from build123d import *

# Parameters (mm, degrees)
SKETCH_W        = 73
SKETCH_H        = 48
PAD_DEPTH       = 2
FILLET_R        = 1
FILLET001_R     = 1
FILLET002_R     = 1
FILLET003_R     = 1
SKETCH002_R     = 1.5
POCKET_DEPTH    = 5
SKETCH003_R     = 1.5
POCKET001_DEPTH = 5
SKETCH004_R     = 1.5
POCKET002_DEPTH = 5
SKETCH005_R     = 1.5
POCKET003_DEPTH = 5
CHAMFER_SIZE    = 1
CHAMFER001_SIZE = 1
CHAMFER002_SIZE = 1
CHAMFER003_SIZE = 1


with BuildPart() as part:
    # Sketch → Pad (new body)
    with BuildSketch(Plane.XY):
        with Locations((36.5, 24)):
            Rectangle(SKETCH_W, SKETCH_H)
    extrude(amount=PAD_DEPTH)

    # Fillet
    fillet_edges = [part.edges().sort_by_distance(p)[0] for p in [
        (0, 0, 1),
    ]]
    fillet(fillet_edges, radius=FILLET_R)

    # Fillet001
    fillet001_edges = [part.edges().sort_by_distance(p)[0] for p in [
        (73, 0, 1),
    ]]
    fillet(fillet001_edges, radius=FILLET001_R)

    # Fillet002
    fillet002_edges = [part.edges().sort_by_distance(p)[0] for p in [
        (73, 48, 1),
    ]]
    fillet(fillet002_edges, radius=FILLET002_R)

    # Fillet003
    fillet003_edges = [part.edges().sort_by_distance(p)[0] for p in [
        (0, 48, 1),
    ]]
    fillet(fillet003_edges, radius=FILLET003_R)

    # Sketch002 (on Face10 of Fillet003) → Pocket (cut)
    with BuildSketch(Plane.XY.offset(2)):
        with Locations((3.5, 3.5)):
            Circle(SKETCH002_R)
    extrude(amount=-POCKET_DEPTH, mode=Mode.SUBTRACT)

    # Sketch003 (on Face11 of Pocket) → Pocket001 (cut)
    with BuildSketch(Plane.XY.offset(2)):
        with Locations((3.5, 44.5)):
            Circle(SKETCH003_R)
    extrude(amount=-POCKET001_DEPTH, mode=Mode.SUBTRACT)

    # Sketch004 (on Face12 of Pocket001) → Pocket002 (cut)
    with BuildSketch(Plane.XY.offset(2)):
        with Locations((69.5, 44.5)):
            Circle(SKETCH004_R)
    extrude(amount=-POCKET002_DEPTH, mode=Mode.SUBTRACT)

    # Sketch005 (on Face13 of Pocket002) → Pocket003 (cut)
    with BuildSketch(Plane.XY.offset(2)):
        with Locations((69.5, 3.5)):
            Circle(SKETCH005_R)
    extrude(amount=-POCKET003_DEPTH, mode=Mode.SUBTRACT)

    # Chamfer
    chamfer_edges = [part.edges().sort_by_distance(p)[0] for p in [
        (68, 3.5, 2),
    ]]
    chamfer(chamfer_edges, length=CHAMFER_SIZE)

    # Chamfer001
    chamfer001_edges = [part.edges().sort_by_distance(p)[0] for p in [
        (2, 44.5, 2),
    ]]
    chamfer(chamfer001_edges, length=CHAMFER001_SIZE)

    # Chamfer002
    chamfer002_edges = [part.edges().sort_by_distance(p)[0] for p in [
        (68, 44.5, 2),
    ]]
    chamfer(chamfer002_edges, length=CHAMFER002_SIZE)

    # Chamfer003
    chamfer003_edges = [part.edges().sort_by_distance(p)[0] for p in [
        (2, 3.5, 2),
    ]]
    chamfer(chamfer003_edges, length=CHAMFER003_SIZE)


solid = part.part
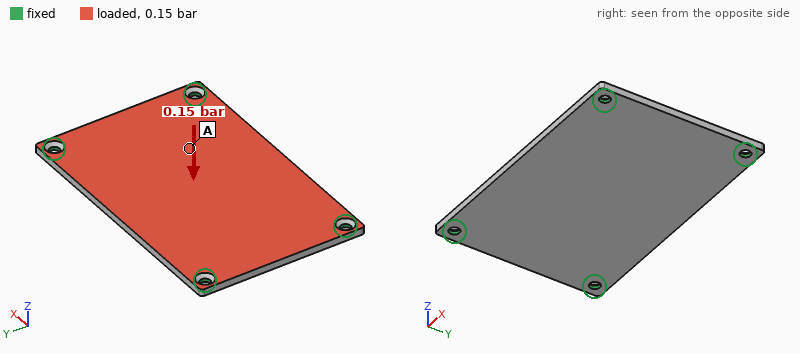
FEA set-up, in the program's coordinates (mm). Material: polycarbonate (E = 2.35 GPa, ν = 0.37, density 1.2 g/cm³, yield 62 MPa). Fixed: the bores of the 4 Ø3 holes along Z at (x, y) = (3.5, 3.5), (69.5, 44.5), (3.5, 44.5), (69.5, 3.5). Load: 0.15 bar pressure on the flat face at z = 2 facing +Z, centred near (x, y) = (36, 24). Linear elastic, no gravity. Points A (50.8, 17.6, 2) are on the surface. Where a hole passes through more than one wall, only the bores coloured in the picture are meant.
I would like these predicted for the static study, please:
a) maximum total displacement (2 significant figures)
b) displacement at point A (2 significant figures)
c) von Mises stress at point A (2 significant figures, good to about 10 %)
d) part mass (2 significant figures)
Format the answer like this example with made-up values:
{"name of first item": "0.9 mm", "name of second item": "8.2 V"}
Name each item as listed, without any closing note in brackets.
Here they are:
{"maximum total displacement": "0.80 mm", "displacement at point A": "0.61 mm", "von Mises stress at point A": "3.4 MPa", "part mass": "8.3 g"}
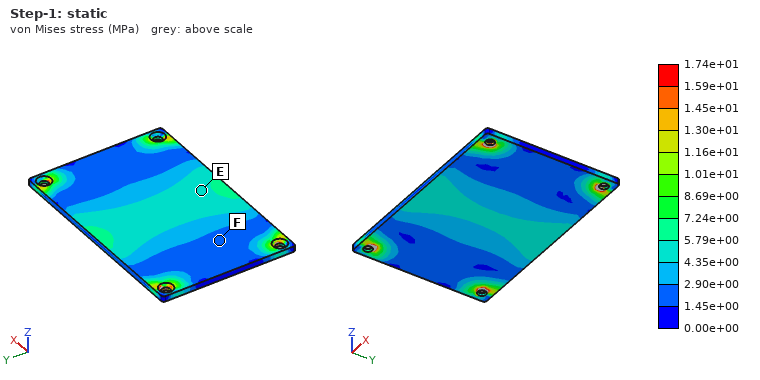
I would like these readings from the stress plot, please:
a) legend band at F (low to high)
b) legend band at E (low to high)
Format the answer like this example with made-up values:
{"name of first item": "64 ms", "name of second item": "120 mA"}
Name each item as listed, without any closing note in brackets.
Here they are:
{"legend band at F": "1.45e+00 to 2.90e+00 MPa", "legend band at E": "4.35e+00 to 5.79e+00 MPa"}
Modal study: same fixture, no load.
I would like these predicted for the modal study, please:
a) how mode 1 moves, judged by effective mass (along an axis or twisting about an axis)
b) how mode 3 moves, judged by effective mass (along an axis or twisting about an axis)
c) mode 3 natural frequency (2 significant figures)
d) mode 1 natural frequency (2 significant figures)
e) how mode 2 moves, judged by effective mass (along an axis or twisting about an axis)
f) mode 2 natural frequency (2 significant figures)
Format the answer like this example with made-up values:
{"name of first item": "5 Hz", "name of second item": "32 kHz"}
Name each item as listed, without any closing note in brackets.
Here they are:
{"how mode 1 moves, judged by effective mass": "along Z", "how mode 3 moves, judged by effective mass": "twisting about Y", "mode 3 natural frequency": "1300 Hz", "mode 1 natural frequency": "510 Hz", "how mode 2 moves, judged by effective mass": "twisting about X", "mode 2 natural frequency": "840 Hz"}
